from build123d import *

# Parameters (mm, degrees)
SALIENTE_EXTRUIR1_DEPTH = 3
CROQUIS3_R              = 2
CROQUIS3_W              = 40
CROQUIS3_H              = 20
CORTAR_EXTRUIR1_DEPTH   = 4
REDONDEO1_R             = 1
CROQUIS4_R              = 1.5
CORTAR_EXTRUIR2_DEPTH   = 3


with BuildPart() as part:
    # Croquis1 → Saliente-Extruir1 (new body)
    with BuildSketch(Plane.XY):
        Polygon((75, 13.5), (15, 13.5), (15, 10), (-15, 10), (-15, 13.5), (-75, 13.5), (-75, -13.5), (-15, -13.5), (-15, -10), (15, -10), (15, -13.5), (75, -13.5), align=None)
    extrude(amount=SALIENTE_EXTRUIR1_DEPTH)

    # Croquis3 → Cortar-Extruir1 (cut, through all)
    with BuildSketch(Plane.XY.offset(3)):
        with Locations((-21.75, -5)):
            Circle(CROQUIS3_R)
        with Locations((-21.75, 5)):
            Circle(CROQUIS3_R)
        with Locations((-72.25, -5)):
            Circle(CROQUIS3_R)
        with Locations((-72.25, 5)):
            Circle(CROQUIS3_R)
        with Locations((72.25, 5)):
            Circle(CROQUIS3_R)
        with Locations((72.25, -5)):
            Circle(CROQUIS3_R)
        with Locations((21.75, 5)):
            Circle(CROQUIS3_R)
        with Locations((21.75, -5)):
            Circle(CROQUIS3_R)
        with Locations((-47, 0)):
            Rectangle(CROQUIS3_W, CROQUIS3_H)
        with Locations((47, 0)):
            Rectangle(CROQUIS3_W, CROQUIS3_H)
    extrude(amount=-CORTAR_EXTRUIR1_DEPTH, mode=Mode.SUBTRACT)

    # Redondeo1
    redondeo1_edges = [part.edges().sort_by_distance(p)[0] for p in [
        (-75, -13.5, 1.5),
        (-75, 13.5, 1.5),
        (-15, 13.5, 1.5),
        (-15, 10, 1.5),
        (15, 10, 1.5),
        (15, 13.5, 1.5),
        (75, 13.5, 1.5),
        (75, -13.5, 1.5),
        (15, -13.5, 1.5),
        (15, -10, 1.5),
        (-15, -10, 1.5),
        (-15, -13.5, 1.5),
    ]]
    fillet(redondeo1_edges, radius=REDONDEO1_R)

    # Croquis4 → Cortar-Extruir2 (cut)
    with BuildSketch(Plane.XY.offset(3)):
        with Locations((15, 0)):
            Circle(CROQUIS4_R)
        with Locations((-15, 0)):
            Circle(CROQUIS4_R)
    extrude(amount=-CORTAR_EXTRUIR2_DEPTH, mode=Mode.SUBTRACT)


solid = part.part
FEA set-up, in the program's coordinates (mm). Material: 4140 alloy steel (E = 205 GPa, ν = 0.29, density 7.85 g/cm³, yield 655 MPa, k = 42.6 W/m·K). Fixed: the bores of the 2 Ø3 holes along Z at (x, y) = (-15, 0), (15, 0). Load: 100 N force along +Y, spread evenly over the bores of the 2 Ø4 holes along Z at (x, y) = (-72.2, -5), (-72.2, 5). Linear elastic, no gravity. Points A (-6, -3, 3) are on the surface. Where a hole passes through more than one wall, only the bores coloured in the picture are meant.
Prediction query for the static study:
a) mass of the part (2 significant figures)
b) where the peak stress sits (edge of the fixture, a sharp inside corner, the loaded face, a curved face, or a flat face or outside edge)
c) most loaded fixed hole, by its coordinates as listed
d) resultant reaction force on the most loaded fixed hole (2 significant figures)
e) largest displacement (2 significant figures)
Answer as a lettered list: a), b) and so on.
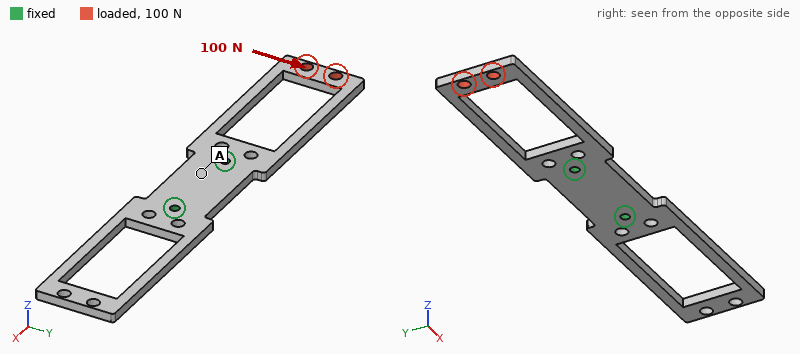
a) 50 g
b) a flat face or outside edge
c) (-15, 0)
d) 260 N
e) 0.19 mm
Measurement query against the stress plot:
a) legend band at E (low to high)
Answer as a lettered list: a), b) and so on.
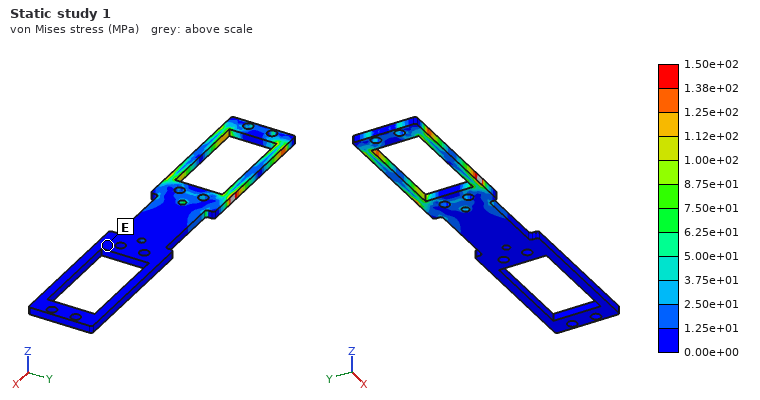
a) 0.00e+00 to 1.25e+01 MPa
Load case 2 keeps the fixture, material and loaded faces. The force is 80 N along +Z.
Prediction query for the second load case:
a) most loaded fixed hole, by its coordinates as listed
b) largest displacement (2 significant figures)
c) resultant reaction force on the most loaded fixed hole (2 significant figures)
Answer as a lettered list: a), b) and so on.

a) (-15, 0)
b) 1.3 mm
c) 120 N
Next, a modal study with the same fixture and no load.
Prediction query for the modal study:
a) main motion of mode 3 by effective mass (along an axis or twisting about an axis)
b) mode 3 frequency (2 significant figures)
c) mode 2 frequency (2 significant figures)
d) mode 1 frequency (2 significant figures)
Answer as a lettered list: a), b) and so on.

a) along Y
b) 1400 Hz
c) 560 Hz
d) 560 Hz
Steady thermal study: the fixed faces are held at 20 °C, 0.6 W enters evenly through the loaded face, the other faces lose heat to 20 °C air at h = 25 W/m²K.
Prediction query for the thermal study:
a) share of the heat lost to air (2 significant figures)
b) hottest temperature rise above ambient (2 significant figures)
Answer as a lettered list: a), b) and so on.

a) 69 %
b) 17 K
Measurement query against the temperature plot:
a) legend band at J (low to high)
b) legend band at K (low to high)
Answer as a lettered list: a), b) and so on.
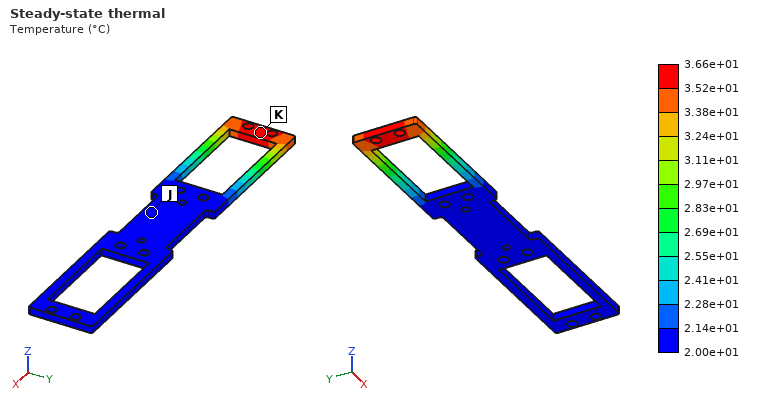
a) 2.00e+01 to 2.14e+01 °C
b) 3.52e+01 to 3.66e+01 °C
